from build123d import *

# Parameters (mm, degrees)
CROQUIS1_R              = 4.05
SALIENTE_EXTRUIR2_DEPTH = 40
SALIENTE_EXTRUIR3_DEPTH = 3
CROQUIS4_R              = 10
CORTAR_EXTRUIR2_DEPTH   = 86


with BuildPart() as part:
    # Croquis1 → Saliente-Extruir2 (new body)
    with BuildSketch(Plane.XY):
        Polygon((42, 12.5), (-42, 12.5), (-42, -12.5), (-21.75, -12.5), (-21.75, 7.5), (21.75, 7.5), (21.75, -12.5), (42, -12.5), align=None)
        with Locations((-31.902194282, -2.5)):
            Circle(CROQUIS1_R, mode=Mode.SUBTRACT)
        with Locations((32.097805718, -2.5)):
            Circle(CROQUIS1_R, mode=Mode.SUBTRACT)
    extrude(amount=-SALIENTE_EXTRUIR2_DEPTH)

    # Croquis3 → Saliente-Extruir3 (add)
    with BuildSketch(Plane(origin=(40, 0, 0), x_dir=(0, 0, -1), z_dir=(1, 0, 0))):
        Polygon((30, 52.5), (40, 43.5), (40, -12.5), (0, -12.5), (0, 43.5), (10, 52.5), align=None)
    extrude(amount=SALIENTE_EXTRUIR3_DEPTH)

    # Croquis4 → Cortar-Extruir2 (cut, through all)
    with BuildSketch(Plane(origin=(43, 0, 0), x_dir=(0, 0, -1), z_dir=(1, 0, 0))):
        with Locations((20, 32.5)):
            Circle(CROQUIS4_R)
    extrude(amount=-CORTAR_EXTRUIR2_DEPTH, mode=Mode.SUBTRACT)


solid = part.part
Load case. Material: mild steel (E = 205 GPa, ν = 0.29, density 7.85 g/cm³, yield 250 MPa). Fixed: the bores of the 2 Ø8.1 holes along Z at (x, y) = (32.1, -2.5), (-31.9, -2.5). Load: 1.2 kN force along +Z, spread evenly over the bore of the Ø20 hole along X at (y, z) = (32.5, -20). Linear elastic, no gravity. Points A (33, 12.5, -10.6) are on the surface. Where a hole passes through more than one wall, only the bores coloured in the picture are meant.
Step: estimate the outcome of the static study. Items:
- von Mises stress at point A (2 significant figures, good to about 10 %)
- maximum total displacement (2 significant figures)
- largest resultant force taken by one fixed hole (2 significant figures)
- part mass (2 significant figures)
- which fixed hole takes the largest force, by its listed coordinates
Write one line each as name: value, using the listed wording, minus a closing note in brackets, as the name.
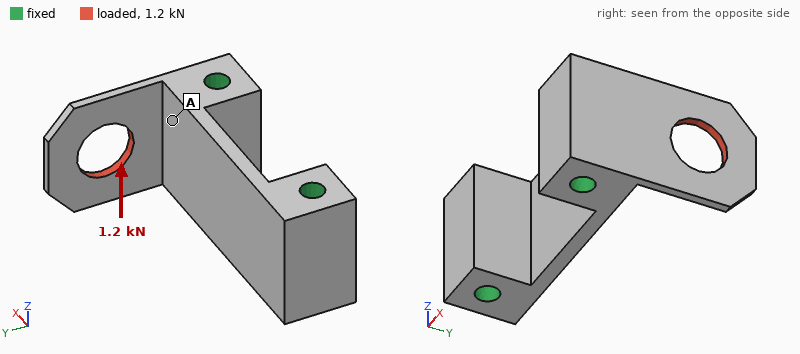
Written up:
von Mises stress at point A: 8.4 MPa
maximum total displacement: 16 µm
largest resultant force taken by one fixed hole: 1.2 kN
part mass: 390 g
which fixed hole takes the largest force, by its listed coordinates: (32.1, -2.5)
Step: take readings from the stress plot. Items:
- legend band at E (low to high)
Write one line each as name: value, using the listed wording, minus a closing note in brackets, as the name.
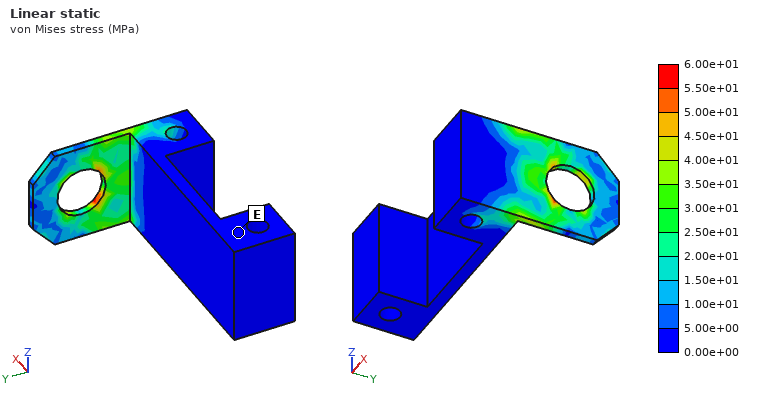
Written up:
legend band at E: 0.00e+00 to 5.00e+00 MPa
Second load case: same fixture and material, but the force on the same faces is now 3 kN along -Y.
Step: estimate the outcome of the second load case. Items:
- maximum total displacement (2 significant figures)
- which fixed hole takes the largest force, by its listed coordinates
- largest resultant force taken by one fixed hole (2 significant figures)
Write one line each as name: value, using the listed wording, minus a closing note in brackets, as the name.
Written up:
maximum total displacement: 13 µm
which fixed hole takes the largest force, by its listed coordinates: (32.1, -2.5)
largest resultant force taken by one fixed hole: 3.0 kN
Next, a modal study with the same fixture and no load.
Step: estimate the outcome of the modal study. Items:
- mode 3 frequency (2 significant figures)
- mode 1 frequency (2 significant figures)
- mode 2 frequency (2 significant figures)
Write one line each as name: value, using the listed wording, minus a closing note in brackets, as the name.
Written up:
mode 3 frequency: 8300 Hz
mode 1 frequency: 1500 Hz
mode 2 frequency: 3800 Hz
